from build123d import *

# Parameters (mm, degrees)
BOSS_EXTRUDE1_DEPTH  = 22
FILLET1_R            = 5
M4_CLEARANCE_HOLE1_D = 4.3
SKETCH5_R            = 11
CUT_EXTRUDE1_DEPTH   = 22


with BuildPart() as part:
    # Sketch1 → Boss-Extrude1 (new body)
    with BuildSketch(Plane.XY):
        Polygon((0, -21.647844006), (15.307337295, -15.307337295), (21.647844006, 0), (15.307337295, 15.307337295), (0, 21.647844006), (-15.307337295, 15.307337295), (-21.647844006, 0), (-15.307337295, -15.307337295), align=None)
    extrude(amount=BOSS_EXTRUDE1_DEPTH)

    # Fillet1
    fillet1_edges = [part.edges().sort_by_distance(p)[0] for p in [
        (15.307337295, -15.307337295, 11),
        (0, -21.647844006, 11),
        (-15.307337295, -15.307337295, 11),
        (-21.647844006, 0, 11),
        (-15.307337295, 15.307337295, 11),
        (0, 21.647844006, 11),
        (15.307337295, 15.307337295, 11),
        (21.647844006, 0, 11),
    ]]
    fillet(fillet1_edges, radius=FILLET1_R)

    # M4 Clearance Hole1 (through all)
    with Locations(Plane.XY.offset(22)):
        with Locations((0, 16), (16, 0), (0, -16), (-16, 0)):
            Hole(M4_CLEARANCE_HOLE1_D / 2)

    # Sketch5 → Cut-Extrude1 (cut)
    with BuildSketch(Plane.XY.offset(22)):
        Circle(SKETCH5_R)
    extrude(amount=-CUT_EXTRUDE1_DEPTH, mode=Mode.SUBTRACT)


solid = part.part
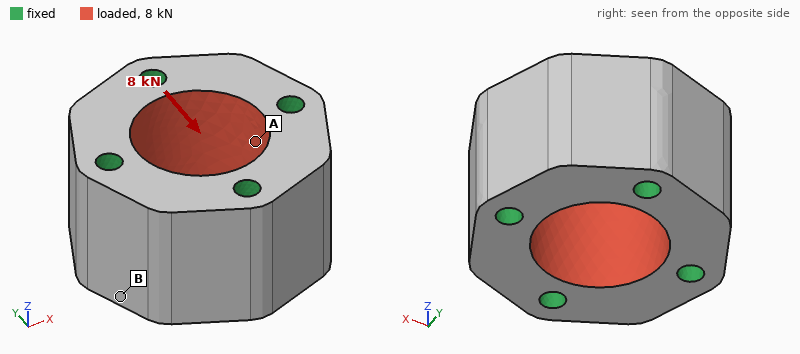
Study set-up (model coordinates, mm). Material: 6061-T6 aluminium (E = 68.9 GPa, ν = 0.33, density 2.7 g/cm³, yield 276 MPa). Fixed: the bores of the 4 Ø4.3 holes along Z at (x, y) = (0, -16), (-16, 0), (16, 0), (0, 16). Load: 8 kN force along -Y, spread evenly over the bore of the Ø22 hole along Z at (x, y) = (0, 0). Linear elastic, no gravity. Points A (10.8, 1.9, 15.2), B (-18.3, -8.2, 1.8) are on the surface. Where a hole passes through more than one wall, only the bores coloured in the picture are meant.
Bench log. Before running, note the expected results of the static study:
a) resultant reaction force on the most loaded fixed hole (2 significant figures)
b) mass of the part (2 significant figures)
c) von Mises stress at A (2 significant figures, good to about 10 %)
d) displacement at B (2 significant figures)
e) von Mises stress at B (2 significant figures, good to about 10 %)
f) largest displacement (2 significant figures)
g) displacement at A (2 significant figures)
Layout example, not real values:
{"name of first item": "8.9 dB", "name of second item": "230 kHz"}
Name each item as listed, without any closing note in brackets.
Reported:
{"resultant reaction force on the most loaded fixed hole": "2.2 kN", "mass of the part": "52 g", "von Mises stress at A": "9.3 MPa", "displacement at B": "0.54 µm", "von Mises stress at B": "3.8 MPa", "largest displacement": "1.6 µm", "displacement at A": "1.1 µm"}
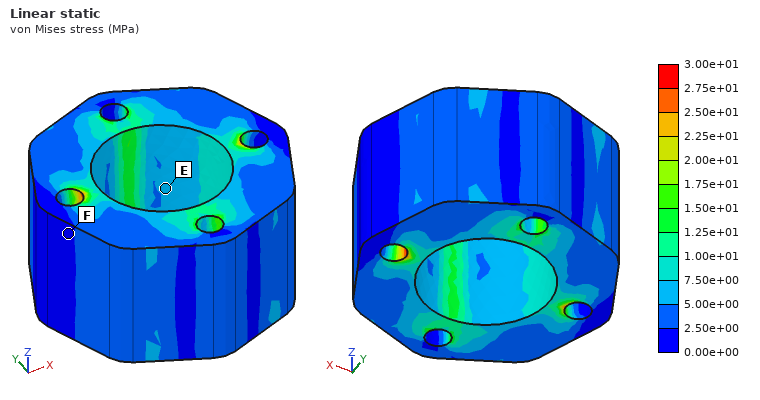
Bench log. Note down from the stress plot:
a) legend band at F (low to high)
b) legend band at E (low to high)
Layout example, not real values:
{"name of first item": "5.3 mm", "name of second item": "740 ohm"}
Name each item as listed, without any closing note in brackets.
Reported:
{"legend band at F": "0.00e+00 to 2.50e+00 MPa", "legend band at E": "5.00e+00 to 7.50e+00 MPa"}
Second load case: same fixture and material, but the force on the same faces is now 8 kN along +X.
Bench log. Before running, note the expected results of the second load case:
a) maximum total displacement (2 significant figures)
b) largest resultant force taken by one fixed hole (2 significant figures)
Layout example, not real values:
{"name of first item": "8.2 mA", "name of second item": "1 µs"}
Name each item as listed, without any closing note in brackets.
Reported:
{"maximum total displacement": "1.6 µm", "largest resultant force taken by one fixed hole": "2.2 kN"}
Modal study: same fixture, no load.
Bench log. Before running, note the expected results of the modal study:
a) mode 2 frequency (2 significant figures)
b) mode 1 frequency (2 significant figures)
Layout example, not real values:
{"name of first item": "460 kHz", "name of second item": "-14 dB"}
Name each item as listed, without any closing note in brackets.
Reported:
{"mode 2 frequency": "56 kHz", "mode 1 frequency": "54 kHz"}
